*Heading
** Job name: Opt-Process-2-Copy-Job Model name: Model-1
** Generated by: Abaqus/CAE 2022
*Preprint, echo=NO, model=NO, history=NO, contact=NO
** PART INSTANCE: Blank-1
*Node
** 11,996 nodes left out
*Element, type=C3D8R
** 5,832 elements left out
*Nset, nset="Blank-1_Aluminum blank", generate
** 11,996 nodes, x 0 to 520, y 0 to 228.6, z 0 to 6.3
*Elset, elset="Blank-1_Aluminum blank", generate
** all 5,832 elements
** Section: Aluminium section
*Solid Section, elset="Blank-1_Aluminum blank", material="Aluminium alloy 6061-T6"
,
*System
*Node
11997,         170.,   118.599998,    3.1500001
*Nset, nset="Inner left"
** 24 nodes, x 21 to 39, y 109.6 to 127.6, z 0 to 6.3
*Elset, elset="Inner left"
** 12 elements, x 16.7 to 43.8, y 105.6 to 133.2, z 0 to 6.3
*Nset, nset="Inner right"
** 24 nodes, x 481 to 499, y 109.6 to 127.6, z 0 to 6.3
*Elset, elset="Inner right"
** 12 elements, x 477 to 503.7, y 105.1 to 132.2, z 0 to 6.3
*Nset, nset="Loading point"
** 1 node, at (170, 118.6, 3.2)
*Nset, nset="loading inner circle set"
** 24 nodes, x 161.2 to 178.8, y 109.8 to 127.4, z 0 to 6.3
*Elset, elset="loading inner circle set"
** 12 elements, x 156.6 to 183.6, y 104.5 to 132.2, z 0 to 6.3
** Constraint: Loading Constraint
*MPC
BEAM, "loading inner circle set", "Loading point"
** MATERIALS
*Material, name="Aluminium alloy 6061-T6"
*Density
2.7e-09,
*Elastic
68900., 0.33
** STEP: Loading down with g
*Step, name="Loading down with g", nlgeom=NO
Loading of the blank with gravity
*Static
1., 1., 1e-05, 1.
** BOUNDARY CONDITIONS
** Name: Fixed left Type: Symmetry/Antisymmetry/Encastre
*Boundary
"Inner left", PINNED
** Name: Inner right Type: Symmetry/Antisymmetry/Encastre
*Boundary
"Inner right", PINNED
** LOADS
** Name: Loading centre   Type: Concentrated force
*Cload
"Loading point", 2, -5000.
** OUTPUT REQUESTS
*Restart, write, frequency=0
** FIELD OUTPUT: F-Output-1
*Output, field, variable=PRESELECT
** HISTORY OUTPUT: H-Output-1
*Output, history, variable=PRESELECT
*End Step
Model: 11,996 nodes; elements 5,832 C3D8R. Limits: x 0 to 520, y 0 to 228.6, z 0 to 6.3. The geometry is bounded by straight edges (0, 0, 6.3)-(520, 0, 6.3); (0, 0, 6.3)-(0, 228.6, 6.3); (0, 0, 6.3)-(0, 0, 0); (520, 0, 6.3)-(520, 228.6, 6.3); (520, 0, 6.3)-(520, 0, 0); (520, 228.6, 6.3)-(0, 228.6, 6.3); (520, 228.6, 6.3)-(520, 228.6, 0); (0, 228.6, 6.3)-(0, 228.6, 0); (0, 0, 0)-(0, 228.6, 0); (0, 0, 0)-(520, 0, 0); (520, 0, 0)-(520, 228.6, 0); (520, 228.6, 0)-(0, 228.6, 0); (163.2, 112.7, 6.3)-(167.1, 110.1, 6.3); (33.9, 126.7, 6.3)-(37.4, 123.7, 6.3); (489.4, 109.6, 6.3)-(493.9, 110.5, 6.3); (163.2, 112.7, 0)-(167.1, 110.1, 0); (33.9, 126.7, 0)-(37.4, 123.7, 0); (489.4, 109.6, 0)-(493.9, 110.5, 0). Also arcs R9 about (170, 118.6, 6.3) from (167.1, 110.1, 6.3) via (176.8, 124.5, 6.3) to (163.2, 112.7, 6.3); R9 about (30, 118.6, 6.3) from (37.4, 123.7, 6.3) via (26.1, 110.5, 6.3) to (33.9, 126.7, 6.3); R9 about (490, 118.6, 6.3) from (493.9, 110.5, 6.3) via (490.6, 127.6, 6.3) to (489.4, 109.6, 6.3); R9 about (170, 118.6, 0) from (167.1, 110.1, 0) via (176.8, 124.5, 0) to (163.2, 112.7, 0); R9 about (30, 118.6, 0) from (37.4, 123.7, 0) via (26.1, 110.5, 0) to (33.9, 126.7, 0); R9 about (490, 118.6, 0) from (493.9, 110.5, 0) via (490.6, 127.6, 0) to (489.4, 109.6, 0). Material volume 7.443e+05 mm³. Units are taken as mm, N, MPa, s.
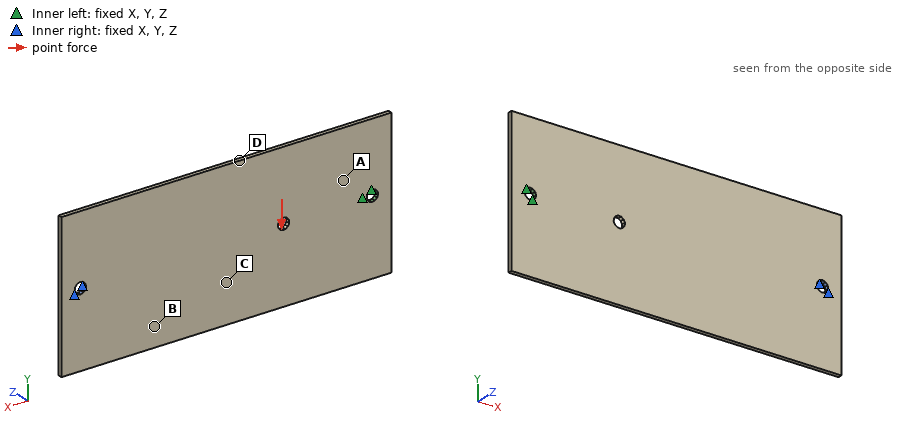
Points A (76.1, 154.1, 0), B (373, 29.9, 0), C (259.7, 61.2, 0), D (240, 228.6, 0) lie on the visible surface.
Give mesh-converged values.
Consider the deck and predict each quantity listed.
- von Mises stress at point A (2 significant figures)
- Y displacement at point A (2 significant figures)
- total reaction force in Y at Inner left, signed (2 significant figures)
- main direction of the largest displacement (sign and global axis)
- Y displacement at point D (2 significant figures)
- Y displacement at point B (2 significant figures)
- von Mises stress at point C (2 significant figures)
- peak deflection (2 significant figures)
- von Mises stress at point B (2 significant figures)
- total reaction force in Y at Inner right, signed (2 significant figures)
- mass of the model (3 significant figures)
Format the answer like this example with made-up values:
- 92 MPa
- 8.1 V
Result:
- 5.6 MPa
- -0.013 mm
- 3500 N
- -Y
- -0.030 mm
- -0.018 mm
- 3.4 MPa
- 0.037 mm
- 2.6 MPa
- 1500 N
- 2.01 kg
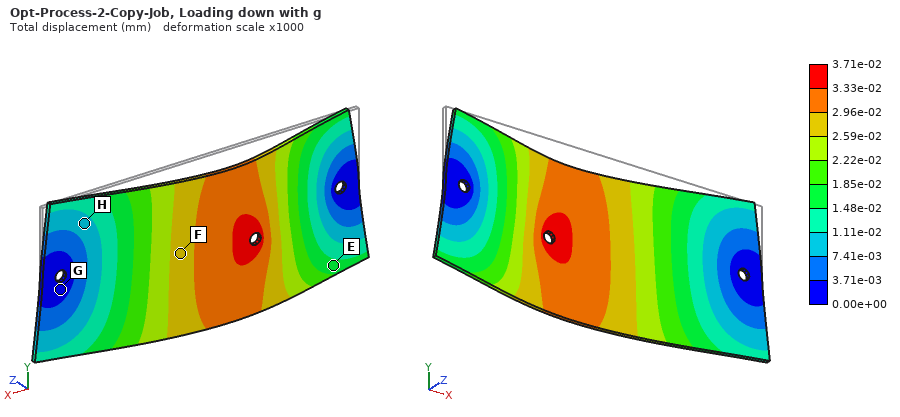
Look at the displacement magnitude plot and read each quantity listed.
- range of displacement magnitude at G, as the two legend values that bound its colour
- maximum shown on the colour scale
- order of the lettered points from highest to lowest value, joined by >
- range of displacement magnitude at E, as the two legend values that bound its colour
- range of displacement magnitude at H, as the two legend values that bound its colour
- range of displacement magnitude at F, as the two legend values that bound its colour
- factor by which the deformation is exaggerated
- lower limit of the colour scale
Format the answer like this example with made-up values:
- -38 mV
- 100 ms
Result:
- 0.00e+00 to 3.71e-03 mm
- 3.71e-02 mm
- F > E > H > G
- 1.48e-02 to 1.85e-02 mm
- 7.41e-03 to 1.11e-02 mm
- 2.59e-02 to 2.96e-02 mm
- 1000
- 0.00e+00 mm
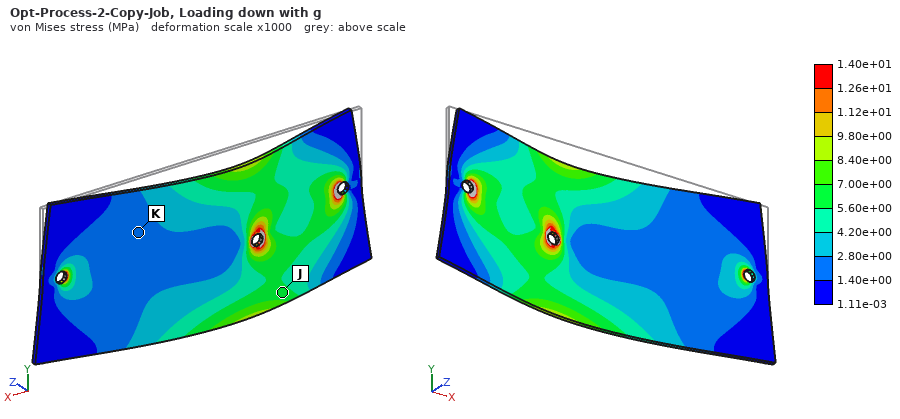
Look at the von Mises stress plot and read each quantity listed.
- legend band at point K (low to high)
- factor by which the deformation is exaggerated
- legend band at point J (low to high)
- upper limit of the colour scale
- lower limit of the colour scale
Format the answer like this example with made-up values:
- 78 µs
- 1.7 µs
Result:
- 1.40e+00 to 2.80e+00 MPa
- 1000
- 5.60e+00 to 7.00e+00 MPa
- 1.40e+01 MPa
- 1.11e-03 MPa
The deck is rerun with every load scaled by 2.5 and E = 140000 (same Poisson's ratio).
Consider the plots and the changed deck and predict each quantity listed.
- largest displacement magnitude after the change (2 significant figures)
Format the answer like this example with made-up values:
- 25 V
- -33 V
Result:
- 0.046 mm
